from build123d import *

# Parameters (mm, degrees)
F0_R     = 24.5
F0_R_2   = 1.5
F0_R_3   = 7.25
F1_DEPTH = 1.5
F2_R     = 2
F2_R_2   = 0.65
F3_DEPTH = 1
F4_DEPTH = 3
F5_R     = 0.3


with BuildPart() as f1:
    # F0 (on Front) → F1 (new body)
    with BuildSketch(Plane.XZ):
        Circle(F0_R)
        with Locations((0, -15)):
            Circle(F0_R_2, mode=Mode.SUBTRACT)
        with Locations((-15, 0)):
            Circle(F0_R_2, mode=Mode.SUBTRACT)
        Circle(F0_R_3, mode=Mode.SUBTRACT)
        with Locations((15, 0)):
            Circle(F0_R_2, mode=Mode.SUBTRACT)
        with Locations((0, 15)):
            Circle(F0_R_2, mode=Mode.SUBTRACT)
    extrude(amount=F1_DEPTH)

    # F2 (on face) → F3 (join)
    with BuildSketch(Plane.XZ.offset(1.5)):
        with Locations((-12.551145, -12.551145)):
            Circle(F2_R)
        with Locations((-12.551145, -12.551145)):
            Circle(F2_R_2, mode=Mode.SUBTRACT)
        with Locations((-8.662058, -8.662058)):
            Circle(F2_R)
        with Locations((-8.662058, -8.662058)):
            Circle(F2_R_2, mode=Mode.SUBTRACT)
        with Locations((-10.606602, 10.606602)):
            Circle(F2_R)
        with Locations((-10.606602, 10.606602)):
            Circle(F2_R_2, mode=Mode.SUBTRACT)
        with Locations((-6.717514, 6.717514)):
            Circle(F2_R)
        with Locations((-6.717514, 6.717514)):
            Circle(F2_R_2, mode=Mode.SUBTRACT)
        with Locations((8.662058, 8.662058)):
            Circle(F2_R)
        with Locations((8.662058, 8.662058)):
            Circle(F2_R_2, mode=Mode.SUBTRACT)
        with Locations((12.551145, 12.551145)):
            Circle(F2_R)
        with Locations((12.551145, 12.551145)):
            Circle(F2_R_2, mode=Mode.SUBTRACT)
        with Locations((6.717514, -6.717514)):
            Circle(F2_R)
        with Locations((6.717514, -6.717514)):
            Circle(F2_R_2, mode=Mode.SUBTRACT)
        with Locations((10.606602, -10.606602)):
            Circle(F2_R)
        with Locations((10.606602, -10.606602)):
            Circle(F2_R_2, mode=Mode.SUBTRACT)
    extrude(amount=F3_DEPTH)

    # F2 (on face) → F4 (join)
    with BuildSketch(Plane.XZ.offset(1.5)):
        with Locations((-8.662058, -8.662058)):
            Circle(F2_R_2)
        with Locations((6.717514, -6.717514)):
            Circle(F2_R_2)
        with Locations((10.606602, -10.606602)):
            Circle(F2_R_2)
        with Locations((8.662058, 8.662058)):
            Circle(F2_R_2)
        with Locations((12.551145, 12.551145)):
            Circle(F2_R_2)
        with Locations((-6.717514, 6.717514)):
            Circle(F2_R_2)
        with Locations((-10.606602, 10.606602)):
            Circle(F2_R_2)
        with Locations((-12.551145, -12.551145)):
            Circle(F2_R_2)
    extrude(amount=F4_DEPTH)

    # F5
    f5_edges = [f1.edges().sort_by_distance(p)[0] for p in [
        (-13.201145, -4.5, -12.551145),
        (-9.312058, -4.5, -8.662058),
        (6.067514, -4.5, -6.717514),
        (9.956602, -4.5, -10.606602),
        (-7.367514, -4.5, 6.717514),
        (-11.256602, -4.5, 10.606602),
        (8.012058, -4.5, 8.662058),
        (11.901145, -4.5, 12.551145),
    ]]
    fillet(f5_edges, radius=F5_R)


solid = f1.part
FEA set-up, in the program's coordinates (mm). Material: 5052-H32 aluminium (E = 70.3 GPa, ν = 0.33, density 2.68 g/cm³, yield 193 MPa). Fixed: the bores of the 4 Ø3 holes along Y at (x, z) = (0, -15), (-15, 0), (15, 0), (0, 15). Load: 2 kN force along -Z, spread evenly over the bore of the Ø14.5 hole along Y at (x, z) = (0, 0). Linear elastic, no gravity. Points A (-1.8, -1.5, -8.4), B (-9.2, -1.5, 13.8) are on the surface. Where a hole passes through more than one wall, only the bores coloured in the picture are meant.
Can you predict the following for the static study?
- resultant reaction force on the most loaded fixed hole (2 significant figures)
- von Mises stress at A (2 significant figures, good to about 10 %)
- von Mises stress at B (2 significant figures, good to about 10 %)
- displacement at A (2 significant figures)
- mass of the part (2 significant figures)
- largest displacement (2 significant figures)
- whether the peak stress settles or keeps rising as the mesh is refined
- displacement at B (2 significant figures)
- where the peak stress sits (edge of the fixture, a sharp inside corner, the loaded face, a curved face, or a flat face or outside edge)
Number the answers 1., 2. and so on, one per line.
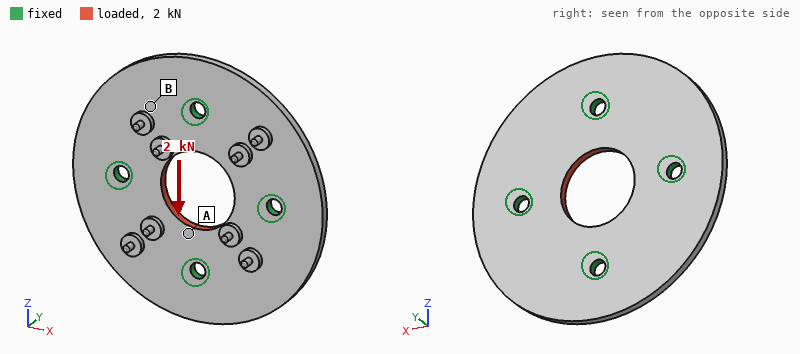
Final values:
1. 580 N
2. 37 MPa
3. 10 MPa
4. 3.6 µm
5. 7.1 g
6. 6.1 µm
7. keeps rising
8. 2.9 µm
9. edge of the fixture
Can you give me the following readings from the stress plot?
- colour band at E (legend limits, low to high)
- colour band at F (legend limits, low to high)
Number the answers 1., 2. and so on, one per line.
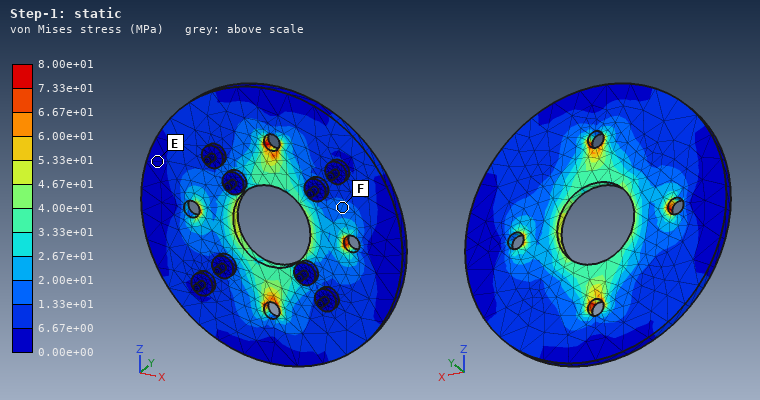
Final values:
1. 0.00e+00 to 6.67e+00 MPa
2. 1.33e+01 to 2.00e+01 MPa
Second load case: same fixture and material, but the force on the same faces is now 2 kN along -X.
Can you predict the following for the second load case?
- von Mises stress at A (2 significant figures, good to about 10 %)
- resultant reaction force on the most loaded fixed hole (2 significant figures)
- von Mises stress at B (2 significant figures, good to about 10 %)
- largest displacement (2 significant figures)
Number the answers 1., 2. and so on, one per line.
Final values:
1. 31 MPa
2. 580 N
3. 11 MPa
4. 6.1 µm
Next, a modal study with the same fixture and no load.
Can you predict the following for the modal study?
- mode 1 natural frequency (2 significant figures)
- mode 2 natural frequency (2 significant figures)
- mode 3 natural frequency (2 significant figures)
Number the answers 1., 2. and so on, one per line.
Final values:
1. 7200 Hz
2. 7700 Hz
3. 7700 Hz
